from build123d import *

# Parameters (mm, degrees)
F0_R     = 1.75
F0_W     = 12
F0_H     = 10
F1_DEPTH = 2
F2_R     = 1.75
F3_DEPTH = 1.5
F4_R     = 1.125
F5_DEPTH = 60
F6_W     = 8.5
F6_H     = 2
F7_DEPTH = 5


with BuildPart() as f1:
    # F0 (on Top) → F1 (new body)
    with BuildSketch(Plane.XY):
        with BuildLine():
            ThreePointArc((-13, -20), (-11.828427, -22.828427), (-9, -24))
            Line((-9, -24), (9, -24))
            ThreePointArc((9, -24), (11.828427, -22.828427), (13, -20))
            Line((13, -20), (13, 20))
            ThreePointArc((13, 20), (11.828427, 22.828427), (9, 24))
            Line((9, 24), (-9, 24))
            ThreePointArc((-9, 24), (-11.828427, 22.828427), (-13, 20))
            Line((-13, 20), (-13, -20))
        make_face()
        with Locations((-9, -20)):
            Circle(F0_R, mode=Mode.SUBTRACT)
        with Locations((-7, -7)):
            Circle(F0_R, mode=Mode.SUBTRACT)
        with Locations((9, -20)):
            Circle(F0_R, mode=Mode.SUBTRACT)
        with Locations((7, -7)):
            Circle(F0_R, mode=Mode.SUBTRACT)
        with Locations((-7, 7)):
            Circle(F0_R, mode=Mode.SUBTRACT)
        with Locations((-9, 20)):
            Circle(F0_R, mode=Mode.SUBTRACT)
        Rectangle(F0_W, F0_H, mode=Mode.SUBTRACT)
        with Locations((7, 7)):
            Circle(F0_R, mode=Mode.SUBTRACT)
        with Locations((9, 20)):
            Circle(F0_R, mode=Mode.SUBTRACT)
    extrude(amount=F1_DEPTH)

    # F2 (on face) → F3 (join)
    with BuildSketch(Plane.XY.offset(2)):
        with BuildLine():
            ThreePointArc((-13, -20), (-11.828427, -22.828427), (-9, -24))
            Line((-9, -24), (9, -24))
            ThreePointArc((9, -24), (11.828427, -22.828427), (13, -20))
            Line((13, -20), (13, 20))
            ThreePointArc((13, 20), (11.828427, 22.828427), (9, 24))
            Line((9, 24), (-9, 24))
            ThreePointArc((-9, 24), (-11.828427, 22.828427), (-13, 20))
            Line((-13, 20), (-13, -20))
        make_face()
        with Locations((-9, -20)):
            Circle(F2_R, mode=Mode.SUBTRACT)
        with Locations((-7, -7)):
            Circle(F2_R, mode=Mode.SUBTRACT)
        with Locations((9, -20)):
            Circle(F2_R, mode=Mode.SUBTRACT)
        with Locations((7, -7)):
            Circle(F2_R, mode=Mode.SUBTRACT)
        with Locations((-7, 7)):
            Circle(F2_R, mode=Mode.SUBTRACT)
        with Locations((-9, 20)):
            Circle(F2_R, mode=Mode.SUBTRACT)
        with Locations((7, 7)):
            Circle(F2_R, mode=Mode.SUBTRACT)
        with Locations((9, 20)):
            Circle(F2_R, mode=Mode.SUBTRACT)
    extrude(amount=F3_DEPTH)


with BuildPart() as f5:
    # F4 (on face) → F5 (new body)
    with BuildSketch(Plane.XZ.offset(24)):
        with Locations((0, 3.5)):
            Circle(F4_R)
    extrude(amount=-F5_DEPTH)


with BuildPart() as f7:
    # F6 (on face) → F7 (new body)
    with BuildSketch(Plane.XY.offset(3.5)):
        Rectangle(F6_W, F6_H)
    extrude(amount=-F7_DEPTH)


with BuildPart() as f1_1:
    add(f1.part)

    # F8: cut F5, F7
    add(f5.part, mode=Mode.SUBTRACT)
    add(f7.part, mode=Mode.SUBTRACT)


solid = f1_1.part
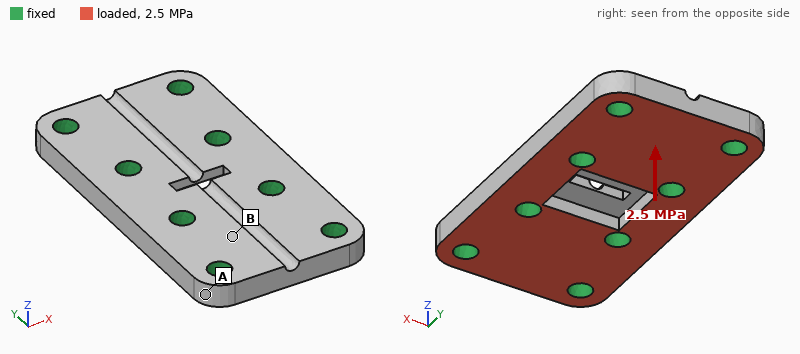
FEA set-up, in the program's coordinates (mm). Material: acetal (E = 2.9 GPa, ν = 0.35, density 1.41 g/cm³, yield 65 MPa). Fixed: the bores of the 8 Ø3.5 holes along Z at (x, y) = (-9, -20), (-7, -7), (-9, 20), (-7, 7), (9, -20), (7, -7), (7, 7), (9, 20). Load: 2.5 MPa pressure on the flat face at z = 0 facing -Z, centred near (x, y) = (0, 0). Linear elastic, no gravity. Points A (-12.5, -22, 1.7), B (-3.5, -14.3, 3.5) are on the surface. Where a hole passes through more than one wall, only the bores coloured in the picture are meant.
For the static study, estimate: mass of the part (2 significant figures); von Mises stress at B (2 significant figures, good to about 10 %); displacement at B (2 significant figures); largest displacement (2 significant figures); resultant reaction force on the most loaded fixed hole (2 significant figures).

5.2 g
6.9 MPa
57 µm
89 µm
350 N
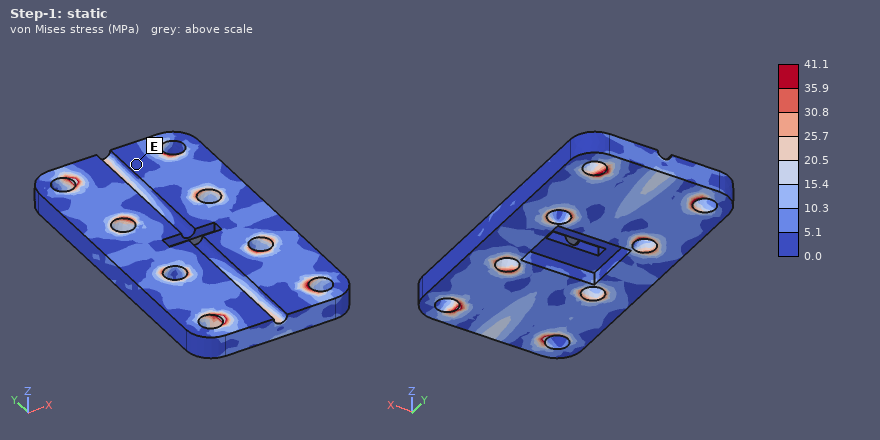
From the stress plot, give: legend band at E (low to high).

0.0 to 5.1 MPa
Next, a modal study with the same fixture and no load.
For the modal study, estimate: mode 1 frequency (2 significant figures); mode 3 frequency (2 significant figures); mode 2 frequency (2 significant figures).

15 kHz
18 kHz
15 kHz
